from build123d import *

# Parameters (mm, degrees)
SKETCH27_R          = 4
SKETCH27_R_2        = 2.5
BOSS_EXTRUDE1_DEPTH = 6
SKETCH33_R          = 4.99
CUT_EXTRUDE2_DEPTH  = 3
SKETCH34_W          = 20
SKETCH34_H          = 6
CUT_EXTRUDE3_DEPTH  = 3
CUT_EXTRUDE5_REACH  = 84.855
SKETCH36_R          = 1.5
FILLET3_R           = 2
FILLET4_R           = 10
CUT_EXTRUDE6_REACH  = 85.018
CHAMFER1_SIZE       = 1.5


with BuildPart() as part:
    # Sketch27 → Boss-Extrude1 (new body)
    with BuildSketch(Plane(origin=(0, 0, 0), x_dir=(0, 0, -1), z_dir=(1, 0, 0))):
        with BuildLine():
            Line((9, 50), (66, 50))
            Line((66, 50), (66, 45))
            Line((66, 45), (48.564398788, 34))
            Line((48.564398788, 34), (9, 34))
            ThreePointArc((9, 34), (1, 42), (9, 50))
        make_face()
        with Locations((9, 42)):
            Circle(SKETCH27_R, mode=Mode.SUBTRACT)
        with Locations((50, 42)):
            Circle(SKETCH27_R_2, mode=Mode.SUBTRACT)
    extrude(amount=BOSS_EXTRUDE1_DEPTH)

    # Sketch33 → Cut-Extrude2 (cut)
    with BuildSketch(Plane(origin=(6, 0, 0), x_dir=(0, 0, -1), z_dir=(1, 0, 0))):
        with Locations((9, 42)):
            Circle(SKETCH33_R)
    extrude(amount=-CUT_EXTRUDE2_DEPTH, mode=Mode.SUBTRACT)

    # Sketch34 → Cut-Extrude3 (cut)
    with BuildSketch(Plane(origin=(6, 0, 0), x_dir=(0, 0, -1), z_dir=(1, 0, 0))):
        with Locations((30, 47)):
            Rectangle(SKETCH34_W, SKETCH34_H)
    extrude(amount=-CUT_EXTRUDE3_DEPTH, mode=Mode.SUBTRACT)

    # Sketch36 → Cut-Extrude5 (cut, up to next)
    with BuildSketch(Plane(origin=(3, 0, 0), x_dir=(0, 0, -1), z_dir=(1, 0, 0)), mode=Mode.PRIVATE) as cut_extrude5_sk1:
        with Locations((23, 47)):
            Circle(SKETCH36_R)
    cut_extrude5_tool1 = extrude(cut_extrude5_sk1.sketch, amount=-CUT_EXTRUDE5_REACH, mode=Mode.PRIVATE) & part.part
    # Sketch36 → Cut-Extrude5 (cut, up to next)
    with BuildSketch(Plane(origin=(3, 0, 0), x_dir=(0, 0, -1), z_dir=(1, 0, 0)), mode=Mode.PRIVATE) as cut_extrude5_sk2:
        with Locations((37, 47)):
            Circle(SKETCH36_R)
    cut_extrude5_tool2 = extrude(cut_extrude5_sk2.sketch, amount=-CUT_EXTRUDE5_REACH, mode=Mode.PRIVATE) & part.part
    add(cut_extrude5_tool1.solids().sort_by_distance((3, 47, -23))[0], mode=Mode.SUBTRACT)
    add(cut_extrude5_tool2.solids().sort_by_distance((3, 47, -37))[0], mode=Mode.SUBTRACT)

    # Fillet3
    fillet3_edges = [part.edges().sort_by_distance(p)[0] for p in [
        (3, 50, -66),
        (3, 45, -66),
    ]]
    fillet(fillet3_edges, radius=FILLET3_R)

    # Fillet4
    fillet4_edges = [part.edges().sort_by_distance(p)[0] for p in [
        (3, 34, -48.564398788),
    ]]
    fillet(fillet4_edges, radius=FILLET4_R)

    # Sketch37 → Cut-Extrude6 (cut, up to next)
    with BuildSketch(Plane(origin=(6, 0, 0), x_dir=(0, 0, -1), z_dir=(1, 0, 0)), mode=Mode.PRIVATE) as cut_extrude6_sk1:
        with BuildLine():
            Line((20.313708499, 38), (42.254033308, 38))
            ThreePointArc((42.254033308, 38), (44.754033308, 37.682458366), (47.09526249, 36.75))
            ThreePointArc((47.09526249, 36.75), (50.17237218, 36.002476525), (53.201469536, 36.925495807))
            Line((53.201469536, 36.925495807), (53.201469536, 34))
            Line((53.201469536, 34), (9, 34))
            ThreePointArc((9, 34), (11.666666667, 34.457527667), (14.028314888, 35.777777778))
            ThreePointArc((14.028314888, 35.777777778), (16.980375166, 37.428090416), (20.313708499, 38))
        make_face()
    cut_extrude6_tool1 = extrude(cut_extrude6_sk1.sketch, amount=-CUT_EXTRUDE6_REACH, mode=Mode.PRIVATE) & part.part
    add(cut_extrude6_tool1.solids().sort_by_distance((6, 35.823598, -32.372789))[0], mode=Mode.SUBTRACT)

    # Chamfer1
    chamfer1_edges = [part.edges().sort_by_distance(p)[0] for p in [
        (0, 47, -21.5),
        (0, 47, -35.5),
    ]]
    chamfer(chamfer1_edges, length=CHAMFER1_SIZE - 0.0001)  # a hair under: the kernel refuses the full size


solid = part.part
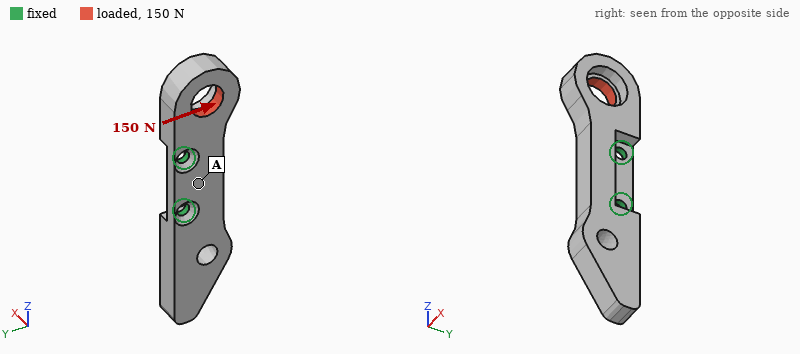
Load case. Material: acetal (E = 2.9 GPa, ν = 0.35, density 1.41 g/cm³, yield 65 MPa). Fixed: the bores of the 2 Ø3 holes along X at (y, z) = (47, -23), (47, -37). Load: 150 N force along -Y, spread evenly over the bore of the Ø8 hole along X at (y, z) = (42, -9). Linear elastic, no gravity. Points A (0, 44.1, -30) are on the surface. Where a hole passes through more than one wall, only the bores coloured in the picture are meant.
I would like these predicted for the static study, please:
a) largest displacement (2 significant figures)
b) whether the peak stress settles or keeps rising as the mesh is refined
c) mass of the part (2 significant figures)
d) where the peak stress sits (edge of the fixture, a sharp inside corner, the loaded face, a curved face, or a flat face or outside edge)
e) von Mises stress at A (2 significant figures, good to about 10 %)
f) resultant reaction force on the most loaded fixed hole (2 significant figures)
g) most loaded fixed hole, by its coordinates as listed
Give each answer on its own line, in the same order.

0.43 mm
keeps rising
5.3 g
edge of the fixture
6.3 MPa
280 N
(47, -23)
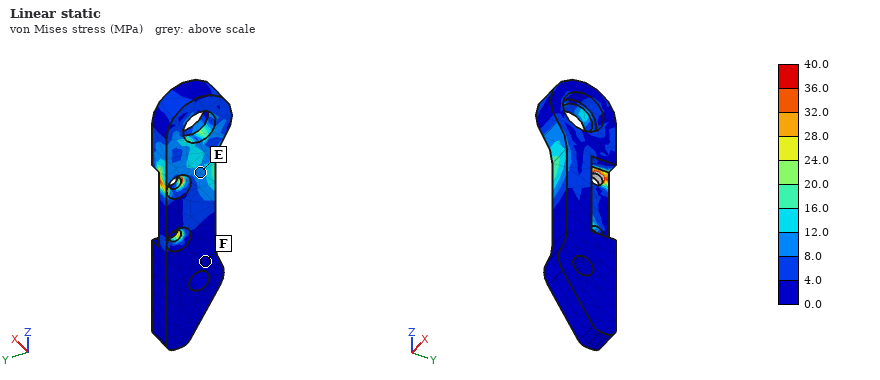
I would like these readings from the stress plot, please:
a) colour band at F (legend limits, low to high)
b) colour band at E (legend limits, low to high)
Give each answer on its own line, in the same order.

0.0 to 4.0 MPa
8.0 to 12.0 MPa
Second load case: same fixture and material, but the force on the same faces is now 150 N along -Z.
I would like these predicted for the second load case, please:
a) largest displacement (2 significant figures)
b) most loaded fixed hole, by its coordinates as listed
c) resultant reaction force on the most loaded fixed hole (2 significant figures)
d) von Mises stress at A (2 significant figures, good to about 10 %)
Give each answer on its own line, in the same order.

0.18 mm
(47, -23)
100 N
3.6 MPa
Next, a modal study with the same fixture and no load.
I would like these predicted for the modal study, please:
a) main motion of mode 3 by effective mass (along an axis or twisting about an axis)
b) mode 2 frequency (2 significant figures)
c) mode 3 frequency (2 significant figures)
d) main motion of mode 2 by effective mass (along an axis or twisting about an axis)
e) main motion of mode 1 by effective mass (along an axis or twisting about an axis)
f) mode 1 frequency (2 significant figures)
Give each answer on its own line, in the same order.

along Y
1600 Hz
2300 Hz
along X
along X
1100 Hz
